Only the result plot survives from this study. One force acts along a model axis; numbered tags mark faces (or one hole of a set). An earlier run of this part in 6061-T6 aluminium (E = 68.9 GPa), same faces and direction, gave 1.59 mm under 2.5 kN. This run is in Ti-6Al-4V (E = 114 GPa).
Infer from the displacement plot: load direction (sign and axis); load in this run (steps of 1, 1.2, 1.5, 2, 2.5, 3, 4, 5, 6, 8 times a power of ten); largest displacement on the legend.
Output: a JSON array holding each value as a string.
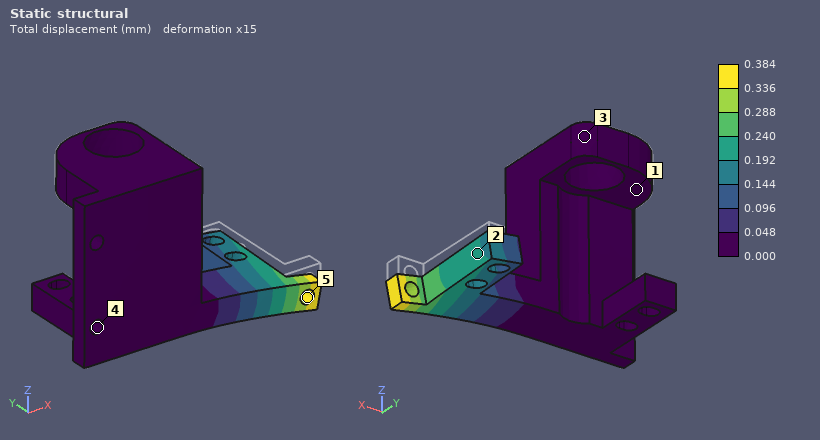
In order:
["-Z", "1 kN", "0.384 mm"]
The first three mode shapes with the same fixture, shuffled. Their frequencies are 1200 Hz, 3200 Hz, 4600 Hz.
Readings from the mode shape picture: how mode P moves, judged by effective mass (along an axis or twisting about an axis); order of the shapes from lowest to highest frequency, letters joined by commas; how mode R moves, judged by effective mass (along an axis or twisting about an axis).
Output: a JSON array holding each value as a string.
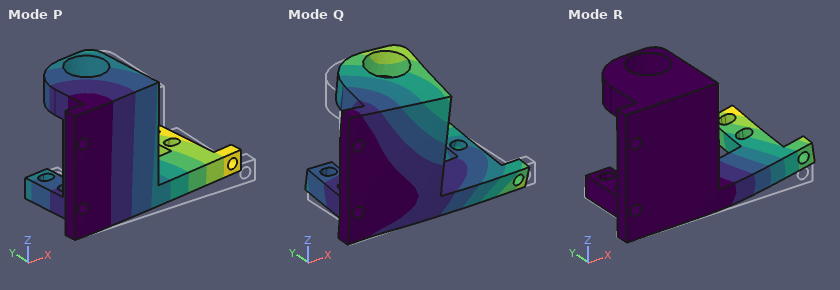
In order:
["along Y", "P, R, Q", "along Z"]
